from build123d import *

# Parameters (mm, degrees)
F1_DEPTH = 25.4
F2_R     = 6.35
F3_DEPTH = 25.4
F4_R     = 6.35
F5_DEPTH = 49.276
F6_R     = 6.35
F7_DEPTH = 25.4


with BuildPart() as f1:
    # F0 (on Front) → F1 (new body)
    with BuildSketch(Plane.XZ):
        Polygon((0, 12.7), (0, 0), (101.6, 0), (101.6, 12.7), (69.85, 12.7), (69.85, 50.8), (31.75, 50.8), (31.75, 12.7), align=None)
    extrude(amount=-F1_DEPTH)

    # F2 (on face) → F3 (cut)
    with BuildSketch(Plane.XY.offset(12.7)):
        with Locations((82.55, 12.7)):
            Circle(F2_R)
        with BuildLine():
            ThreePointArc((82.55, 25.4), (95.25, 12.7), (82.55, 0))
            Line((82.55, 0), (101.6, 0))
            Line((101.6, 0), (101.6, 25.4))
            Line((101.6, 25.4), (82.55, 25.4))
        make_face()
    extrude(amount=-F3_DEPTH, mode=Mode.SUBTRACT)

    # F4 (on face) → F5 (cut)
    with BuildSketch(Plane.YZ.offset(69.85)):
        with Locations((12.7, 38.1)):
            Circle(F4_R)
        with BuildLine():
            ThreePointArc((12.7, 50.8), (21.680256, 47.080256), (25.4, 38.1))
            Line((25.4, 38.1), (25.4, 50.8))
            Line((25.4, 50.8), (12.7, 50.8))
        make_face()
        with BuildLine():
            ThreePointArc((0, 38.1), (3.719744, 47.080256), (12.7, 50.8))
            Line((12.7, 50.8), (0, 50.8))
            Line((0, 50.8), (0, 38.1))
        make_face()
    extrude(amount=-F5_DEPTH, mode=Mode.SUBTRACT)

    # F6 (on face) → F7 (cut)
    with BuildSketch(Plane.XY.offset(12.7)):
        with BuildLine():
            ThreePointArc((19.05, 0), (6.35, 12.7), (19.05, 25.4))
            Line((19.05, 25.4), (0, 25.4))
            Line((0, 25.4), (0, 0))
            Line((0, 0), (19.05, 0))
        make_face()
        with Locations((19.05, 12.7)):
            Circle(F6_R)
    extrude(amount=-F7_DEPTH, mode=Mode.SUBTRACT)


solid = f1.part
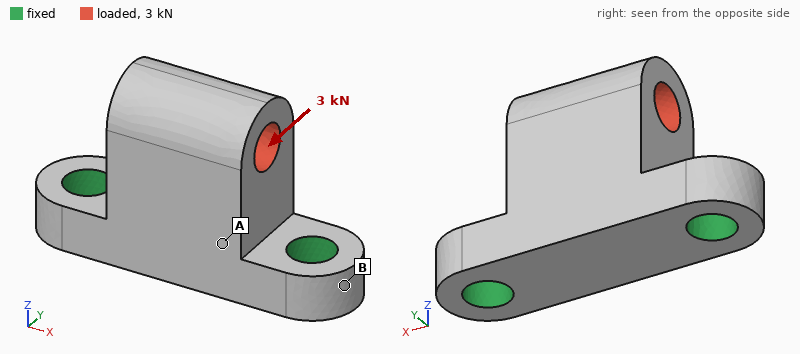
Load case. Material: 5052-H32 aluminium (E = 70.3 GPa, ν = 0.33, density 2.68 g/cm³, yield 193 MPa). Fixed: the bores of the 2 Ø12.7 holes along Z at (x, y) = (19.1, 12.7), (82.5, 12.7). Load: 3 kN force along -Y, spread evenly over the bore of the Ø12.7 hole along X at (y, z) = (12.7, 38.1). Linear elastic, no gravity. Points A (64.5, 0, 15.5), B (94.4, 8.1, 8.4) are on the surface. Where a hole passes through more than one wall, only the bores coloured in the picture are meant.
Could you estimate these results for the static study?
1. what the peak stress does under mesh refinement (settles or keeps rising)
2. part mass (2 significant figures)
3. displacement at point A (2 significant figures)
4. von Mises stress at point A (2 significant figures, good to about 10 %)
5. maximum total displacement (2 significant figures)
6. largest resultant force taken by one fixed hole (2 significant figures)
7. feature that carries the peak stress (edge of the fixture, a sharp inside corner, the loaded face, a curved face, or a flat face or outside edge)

keeps rising
140 g
28 µm
19 MPa
90 µm
1.5 kN
edge of the fixture
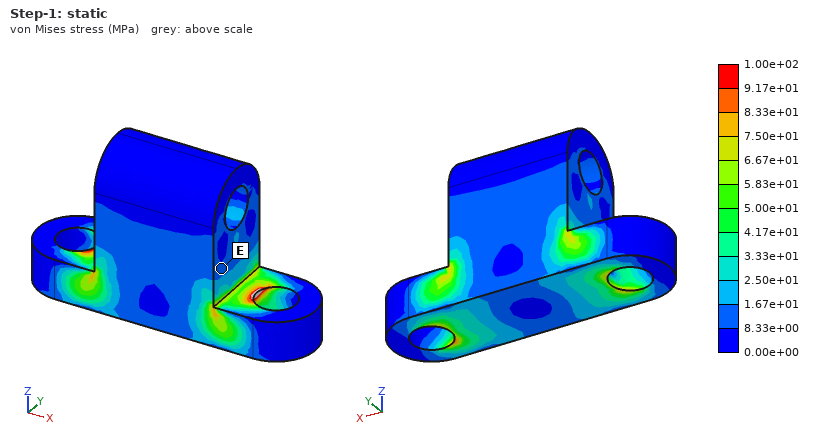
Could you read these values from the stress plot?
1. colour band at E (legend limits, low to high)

8.33e+00 to 1.67e+01 MPa
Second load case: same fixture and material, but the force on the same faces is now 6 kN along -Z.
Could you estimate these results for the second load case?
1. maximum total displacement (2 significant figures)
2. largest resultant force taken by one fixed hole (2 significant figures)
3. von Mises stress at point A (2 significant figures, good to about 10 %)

13 µm
3.2 kN
11 MPa
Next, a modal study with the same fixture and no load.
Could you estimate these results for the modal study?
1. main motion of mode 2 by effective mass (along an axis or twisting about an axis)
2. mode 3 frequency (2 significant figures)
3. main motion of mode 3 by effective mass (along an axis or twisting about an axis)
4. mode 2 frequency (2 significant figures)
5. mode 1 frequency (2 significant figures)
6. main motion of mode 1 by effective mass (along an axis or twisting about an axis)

along X
12 kHz
along Z
10 kHz
4700 Hz
along Y
